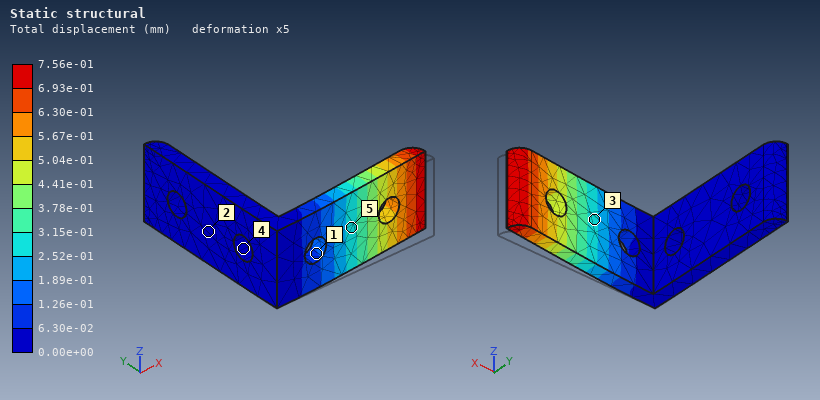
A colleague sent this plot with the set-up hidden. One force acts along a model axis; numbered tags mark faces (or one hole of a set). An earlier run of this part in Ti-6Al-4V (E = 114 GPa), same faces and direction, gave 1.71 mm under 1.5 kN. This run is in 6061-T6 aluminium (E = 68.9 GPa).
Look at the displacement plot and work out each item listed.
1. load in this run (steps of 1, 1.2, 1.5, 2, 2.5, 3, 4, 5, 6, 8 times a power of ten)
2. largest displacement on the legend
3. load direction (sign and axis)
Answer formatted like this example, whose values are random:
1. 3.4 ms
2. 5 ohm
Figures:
1. 400 N
2. 7.56e-01 mm
3. +Y
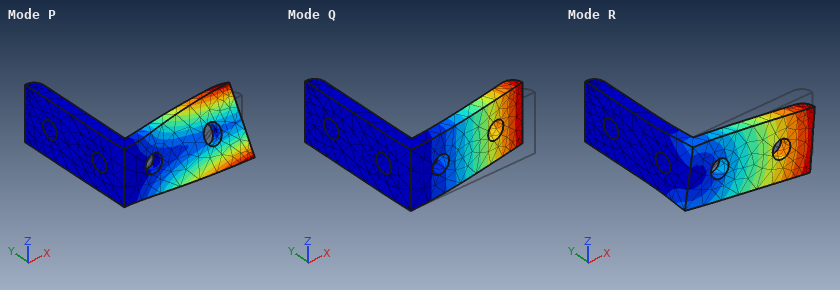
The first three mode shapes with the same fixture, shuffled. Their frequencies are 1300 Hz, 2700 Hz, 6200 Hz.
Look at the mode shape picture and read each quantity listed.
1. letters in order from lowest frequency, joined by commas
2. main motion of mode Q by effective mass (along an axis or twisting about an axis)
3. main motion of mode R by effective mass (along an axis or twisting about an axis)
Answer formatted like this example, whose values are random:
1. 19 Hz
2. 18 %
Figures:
1. Q, R, P
2. along Y
3. along Z
